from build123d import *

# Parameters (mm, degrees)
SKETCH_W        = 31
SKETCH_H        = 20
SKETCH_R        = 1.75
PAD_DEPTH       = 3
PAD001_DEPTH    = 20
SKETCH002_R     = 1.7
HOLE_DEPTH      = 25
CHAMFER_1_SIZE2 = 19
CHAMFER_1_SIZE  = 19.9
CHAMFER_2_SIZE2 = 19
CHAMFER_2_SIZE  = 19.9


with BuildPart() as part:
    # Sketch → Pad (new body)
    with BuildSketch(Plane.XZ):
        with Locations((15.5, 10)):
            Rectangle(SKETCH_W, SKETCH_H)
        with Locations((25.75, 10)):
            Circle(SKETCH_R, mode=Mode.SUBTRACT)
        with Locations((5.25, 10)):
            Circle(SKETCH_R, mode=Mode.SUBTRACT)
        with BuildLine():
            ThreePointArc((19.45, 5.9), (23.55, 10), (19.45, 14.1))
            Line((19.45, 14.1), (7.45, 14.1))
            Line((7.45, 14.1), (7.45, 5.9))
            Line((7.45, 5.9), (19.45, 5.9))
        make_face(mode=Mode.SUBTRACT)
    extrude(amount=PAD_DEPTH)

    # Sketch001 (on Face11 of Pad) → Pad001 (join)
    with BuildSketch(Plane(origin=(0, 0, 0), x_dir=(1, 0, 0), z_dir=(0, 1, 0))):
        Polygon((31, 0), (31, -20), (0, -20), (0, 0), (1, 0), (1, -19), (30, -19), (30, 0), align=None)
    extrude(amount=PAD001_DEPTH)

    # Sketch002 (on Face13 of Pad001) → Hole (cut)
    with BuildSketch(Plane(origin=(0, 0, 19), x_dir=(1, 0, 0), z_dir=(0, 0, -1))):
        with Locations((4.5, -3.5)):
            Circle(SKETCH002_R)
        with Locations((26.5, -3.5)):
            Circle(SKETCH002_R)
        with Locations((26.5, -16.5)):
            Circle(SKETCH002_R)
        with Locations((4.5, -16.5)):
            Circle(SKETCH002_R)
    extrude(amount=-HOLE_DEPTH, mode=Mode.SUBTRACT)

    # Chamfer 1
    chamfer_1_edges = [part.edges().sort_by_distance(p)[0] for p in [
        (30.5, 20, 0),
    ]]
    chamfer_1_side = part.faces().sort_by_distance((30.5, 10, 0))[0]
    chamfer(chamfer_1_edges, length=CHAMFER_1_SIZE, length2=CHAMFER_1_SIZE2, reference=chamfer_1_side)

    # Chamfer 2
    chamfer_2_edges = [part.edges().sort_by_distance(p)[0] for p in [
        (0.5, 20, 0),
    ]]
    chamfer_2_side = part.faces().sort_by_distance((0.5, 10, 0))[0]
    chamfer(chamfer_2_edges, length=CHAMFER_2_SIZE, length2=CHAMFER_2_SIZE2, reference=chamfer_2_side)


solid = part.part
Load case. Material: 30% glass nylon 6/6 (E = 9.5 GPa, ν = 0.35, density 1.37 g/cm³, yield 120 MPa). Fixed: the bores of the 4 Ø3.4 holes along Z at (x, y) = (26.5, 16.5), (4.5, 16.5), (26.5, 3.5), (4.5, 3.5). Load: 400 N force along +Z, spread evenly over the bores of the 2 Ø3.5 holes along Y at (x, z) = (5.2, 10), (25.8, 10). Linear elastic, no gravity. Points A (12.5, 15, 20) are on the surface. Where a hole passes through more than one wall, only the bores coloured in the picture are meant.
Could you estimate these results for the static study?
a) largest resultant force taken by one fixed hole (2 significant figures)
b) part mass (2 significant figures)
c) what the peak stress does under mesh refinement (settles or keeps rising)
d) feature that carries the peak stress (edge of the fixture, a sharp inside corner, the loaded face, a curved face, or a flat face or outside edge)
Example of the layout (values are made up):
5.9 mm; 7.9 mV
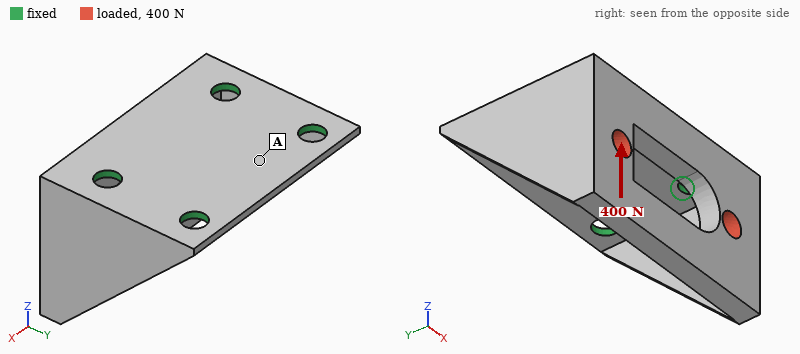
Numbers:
250 N; 3.3 g; keeps rising; edge of the fixture
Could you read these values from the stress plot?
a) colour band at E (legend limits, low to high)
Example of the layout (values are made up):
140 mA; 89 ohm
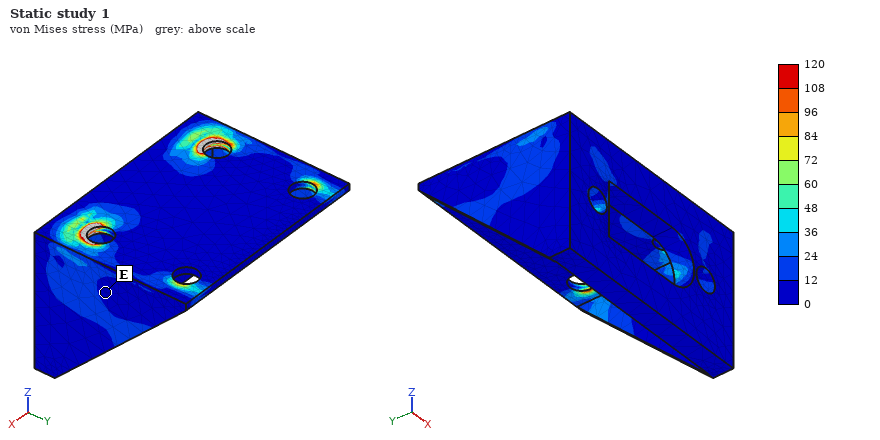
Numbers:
0 to 12 MPa
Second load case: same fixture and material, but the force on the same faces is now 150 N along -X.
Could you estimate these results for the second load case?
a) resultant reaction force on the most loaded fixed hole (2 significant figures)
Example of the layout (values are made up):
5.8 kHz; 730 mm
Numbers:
100 N
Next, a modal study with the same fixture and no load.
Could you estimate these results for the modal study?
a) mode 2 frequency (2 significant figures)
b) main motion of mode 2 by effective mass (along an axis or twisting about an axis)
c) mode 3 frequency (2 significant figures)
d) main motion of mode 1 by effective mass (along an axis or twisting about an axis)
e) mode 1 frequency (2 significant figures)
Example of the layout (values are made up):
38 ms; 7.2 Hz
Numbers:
4100 Hz; along X; 6600 Hz; along Y; 3200 Hz
